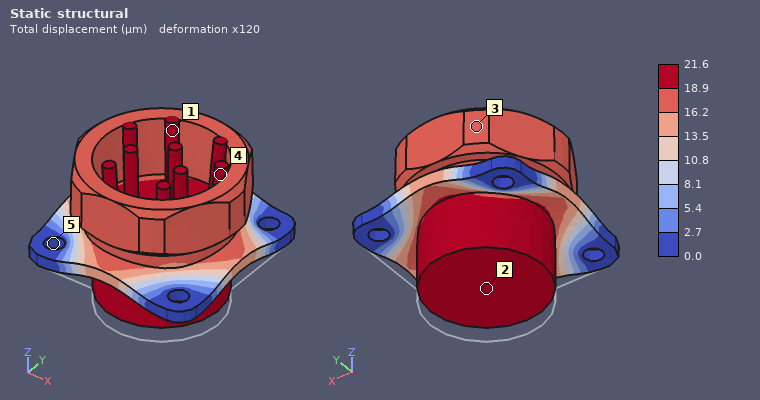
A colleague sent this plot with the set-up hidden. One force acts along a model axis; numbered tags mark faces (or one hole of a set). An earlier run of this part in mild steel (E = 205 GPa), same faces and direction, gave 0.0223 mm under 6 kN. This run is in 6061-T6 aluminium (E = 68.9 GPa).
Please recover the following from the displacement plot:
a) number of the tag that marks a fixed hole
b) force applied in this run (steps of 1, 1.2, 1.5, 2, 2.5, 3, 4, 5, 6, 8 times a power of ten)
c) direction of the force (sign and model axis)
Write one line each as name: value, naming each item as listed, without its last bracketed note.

number of the tag that marks a fixed hole: 5
force applied in this run: 2 kN
direction of the force: +Z
